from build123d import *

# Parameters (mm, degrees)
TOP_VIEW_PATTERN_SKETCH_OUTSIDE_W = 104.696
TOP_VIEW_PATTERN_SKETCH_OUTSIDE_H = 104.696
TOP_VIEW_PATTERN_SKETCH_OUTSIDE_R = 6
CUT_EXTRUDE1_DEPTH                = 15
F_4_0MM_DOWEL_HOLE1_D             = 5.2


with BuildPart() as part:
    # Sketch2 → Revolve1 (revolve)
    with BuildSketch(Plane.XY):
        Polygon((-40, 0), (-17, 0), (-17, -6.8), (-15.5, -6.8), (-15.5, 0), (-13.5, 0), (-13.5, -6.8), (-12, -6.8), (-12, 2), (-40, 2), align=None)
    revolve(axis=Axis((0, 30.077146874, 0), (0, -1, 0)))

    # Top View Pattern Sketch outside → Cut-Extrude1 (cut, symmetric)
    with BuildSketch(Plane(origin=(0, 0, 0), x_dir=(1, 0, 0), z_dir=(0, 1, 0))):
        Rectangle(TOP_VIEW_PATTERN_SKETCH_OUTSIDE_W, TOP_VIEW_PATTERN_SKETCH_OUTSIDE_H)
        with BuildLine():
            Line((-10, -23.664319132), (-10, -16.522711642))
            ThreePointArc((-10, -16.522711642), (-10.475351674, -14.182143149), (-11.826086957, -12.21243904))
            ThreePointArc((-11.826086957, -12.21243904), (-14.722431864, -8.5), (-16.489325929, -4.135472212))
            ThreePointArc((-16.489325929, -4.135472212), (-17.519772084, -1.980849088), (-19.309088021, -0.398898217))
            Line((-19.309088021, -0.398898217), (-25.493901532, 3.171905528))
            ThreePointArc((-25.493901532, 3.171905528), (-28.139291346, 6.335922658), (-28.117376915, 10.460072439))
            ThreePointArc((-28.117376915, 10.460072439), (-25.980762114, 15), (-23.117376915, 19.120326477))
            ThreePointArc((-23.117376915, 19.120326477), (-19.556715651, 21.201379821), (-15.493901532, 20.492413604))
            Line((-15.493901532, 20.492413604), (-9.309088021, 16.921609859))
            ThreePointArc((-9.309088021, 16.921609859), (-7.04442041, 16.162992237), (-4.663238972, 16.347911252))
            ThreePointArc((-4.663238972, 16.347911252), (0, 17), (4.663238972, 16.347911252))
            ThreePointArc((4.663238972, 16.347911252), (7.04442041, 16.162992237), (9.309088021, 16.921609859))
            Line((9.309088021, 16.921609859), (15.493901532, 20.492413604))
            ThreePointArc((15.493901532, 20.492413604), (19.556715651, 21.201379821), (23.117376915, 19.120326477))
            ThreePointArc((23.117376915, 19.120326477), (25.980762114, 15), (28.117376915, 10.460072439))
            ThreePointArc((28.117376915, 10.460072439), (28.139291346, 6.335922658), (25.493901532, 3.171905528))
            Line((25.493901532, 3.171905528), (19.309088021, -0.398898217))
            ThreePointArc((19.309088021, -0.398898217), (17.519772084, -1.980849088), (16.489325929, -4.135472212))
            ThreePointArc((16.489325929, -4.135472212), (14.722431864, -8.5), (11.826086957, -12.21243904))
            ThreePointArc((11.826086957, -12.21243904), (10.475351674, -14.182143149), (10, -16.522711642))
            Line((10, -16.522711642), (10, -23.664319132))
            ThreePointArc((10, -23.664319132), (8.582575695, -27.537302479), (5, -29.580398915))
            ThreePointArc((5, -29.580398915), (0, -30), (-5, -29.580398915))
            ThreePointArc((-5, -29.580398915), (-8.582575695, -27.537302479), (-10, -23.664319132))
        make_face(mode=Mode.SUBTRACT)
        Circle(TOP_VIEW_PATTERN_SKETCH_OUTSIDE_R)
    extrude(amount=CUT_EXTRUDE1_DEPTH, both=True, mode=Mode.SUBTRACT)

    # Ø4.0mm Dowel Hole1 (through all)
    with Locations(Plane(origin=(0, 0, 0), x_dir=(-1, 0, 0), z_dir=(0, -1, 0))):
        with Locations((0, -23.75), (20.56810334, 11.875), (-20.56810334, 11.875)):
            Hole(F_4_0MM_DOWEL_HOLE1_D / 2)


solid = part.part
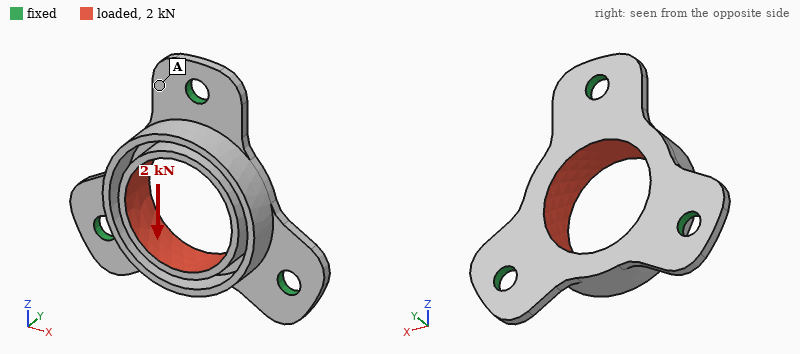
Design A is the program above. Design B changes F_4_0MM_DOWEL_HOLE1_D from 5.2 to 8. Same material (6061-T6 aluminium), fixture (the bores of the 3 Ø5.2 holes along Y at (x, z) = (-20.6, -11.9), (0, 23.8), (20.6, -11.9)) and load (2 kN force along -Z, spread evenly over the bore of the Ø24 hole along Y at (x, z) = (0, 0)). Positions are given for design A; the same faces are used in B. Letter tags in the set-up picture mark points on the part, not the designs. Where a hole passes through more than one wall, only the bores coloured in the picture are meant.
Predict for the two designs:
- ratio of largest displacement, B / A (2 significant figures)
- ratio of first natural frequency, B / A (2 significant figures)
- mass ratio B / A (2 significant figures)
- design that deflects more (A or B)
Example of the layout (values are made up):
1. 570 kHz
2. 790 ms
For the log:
1. 0.72
2. 1.2
3. 0.96
4. A
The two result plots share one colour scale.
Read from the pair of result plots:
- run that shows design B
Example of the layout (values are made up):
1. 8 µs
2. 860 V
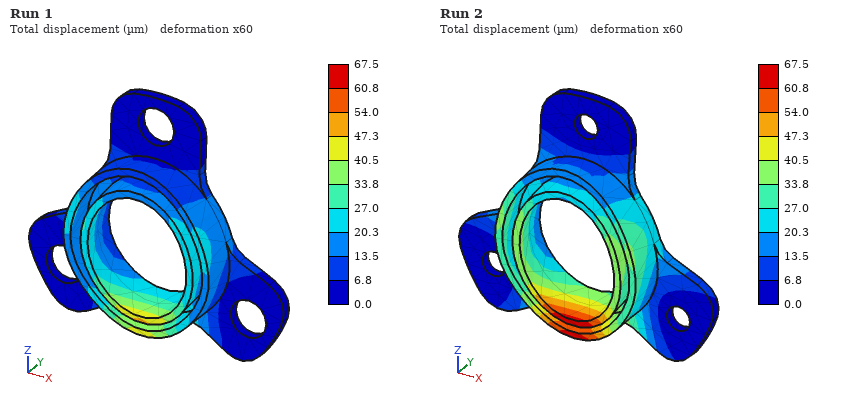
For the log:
1. Run 1
